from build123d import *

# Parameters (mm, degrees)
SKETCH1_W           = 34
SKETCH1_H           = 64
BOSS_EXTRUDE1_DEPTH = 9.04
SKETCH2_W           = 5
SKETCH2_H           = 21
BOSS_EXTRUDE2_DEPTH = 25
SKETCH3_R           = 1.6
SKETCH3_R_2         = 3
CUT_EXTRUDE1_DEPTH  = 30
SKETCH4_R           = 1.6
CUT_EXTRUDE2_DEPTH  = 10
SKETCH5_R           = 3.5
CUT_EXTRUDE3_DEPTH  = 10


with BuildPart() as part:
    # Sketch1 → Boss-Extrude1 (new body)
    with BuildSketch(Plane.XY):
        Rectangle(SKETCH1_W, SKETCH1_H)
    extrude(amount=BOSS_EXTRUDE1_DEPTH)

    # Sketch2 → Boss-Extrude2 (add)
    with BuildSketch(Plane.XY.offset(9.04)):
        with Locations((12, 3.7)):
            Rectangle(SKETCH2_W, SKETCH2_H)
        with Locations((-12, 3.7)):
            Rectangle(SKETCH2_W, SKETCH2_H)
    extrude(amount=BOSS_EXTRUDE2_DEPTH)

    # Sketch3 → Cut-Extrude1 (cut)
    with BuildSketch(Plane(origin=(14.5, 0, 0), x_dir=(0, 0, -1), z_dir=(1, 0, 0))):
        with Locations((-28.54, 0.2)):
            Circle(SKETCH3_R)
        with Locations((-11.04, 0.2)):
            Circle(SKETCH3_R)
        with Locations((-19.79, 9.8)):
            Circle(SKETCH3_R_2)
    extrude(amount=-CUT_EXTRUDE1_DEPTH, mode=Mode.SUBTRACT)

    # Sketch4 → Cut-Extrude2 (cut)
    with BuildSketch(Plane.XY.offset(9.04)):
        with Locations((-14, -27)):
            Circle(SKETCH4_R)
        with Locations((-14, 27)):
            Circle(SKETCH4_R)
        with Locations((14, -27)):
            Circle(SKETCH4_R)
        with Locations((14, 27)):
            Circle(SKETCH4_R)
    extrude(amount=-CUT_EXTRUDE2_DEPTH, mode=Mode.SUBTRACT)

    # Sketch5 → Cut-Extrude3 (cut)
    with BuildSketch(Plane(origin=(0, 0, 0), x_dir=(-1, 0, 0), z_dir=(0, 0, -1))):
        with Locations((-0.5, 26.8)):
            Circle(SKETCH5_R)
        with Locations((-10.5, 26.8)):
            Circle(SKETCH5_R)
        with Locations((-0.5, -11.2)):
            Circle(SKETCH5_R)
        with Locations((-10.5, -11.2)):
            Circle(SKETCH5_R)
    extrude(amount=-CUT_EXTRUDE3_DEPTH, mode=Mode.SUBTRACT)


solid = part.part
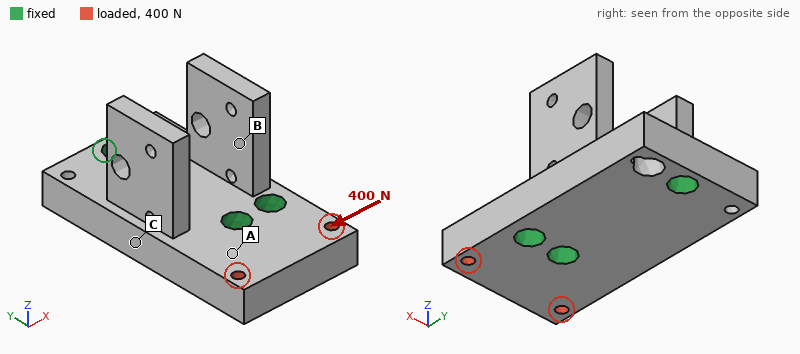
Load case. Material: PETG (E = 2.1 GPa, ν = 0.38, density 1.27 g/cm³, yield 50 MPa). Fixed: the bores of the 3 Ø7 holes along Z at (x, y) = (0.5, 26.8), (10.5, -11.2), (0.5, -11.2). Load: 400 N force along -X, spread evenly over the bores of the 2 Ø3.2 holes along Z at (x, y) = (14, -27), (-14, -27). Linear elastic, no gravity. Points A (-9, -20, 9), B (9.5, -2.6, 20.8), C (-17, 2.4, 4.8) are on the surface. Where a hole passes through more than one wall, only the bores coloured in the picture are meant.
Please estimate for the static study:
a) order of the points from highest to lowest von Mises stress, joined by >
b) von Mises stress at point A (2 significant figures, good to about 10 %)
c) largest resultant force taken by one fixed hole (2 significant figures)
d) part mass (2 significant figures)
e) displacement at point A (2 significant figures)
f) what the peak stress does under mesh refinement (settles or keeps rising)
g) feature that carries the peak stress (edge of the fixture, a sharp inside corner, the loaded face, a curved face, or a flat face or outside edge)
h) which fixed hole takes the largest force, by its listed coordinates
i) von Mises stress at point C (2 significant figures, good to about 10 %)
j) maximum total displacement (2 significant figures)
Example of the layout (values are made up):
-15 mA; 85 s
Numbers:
A > C > B; 2.3 MPa; 340 N; 29 g; 28 µm; keeps rising; edge of the fixture; (0.5, -11.2); 1.2 MPa; 67 µm
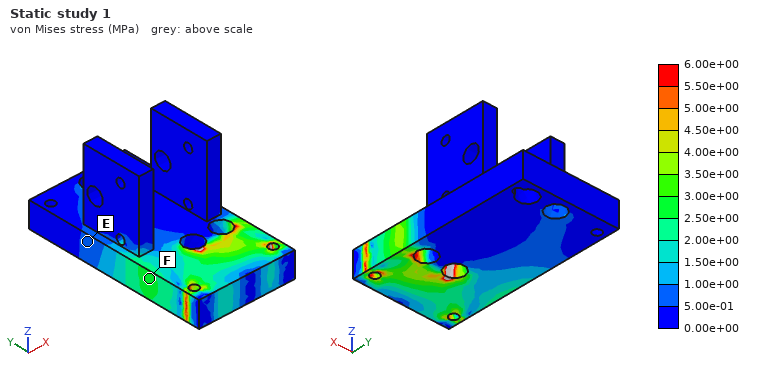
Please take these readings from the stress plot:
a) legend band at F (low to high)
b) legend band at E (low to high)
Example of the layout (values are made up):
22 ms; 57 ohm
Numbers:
2.50e+00 to 3.00e+00 MPa; 5.00e-01 to 1.00e+00 MPa
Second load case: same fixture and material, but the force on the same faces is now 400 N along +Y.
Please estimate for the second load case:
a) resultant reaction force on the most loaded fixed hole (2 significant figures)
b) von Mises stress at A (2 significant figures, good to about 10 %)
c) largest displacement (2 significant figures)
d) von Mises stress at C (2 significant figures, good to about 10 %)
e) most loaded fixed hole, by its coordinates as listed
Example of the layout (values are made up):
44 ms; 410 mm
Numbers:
210 N; 1.6 MPa; 40 µm; 0.74 MPa; (0.5, -11.2)
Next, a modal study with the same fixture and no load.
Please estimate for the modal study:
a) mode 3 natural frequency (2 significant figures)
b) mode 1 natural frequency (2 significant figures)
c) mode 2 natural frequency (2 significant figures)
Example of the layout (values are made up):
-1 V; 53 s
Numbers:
3100 Hz; 1300 Hz; 1300 Hz
